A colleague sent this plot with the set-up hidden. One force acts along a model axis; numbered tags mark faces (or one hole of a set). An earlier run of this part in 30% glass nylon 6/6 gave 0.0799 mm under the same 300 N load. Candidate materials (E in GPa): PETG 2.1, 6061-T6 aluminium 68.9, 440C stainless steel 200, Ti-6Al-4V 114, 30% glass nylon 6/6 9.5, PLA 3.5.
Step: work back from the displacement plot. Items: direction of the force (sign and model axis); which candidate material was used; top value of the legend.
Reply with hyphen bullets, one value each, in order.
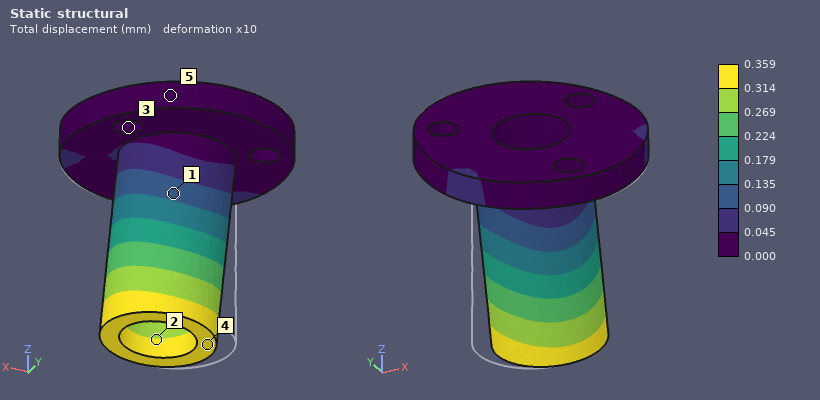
- +X
- PETG
- 0.359 mm
